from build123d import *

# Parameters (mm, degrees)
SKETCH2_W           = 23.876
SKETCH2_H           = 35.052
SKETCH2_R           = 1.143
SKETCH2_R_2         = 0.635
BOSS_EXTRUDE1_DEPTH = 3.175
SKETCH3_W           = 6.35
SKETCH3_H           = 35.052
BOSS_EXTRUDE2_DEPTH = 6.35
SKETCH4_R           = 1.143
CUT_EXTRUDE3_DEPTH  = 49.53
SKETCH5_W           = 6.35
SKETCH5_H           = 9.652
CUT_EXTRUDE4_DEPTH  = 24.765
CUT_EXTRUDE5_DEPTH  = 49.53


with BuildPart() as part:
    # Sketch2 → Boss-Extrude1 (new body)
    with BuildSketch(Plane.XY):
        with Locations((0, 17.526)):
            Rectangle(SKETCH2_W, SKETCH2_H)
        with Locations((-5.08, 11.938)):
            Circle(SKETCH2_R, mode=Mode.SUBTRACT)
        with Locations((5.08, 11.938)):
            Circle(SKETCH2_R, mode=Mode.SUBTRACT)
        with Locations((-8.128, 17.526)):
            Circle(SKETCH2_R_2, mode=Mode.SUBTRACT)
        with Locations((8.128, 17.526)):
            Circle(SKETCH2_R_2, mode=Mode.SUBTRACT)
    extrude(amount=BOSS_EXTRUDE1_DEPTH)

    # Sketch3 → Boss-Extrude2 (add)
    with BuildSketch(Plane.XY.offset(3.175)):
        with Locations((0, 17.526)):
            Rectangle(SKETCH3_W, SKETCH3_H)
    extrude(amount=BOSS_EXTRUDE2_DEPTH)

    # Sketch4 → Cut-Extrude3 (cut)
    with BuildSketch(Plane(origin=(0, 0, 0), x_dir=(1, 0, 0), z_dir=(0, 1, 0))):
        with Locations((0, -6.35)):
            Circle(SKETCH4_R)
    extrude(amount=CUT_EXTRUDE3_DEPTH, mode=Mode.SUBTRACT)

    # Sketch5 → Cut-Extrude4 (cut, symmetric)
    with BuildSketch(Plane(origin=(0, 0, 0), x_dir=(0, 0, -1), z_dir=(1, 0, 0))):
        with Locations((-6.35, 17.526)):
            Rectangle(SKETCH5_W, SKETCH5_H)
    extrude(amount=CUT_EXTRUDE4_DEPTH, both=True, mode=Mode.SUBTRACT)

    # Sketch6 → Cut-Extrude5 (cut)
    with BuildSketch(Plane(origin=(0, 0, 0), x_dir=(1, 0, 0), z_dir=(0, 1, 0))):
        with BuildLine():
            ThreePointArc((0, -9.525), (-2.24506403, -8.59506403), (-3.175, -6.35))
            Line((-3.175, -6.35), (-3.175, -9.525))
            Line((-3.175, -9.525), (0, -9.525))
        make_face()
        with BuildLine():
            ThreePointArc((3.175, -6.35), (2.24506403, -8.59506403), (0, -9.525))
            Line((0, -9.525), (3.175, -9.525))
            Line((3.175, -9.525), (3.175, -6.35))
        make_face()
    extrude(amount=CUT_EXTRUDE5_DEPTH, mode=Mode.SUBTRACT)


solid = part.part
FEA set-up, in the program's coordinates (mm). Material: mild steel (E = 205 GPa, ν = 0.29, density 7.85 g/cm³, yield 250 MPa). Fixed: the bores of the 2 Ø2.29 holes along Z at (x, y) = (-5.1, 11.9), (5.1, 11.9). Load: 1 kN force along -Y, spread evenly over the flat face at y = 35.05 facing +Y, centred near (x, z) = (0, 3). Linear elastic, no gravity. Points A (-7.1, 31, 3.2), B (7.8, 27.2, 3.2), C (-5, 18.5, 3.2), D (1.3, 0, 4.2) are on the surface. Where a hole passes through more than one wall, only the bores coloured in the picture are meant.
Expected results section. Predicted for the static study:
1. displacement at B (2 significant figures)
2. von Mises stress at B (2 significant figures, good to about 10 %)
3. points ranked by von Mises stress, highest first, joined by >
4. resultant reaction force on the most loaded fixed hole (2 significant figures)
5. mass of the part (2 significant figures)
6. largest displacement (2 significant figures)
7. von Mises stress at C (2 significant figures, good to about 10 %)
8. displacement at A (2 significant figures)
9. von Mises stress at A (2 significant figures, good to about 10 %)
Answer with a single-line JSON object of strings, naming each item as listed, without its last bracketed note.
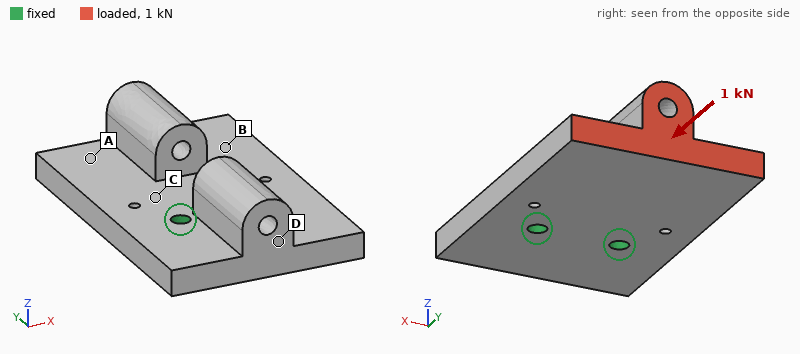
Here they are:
{"displacement at B": "12 µm", "von Mises stress at B": "21 MPa", "points ranked by von Mises stress, highest first, joined by >": "C > B > A > D", "resultant reaction force on the most loaded fixed hole": "500 N", "mass of the part": "27 g", "largest displacement": "26 µm", "von Mises stress at C": "48 MPa", "displacement at A": "17 µm", "von Mises stress at A": "13 MPa"}
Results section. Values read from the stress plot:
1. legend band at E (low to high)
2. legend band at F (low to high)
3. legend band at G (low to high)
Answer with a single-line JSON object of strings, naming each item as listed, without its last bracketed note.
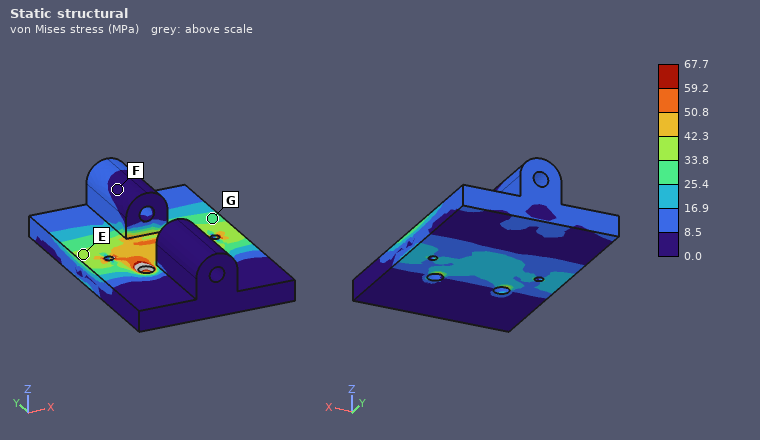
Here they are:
{"legend band at E": "33.8 to 42.3 MPa", "legend band at F": "0.0 to 8.5 MPa", "legend band at G": "25.4 to 33.8 MPa"}
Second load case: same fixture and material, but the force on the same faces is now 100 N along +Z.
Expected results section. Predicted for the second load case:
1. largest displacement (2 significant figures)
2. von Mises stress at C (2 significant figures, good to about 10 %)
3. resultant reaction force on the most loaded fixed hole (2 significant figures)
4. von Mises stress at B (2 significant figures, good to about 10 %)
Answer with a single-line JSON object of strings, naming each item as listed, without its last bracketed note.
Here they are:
{"largest displacement": "34 µm", "von Mises stress at C": "40 MPa", "resultant reaction force on the most loaded fixed hole": "50 N", "von Mises stress at B": "12 MPa"}
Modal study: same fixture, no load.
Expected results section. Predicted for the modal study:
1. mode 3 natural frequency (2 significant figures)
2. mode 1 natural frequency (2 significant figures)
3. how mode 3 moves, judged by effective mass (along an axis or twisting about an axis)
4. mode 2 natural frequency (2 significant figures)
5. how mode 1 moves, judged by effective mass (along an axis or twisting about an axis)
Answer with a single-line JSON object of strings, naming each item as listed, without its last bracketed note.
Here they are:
{"mode 3 natural frequency": "15 kHz", "mode 1 natural frequency": "3900 Hz", "how mode 3 moves, judged by effective mass": "along Z", "mode 2 natural frequency": "10 kHz", "how mode 1 moves, judged by effective mass": "along Z"}
